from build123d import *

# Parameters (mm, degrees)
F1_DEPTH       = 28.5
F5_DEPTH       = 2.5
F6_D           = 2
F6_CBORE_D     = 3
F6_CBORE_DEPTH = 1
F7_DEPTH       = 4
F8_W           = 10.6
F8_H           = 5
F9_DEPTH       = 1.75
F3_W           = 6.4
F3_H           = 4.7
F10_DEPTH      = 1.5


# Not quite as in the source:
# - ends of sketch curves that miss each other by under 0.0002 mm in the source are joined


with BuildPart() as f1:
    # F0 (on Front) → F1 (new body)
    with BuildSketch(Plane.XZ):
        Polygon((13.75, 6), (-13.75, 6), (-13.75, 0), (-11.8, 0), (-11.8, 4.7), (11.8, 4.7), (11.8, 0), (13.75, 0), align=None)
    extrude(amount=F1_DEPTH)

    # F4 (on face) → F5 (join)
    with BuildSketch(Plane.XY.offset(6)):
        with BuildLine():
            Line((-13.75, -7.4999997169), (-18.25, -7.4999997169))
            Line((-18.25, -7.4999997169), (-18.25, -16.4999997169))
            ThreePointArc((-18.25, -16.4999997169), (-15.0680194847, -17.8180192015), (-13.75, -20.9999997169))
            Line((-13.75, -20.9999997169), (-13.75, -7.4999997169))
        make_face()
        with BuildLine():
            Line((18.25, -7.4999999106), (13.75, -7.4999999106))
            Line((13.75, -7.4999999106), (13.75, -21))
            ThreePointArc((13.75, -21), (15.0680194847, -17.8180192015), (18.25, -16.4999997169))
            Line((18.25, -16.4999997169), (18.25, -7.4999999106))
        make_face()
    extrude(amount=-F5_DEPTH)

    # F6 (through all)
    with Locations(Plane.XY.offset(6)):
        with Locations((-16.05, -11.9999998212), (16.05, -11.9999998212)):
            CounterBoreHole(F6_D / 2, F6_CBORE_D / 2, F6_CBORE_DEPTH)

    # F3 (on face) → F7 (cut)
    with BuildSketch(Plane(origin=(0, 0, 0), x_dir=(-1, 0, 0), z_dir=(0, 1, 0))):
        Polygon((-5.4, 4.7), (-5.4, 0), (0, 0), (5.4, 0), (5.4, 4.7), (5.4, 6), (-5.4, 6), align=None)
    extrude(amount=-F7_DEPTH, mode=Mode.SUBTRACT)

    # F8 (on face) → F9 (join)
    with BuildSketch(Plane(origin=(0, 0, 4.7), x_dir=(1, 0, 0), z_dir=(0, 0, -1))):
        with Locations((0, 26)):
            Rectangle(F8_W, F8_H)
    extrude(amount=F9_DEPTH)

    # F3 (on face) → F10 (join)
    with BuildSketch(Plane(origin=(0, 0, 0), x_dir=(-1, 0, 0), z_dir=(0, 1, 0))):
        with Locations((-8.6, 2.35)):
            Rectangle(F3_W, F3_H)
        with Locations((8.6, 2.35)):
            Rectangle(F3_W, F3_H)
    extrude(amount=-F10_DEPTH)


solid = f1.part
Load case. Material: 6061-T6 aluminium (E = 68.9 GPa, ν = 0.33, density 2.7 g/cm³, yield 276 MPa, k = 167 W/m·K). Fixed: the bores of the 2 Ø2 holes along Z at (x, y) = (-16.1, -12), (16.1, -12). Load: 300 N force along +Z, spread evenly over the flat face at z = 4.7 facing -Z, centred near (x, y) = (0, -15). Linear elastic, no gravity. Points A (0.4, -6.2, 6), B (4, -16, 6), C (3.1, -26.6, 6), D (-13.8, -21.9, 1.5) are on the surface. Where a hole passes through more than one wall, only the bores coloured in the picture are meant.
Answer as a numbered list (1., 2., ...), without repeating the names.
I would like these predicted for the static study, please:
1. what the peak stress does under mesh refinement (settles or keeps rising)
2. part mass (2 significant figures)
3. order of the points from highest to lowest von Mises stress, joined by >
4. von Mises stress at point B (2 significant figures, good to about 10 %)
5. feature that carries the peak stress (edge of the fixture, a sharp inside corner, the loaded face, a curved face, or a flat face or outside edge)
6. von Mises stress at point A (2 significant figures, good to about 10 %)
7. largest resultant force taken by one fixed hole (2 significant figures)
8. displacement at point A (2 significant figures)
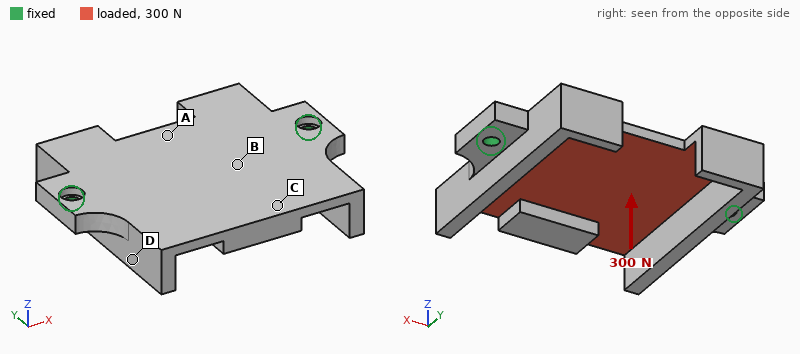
1. keeps rising
2. 5.0 g
3. A > B > C > D
4. 49 MPa
5. edge of the fixture
6. 70 MPa
7. 310 N
8. 61 µm
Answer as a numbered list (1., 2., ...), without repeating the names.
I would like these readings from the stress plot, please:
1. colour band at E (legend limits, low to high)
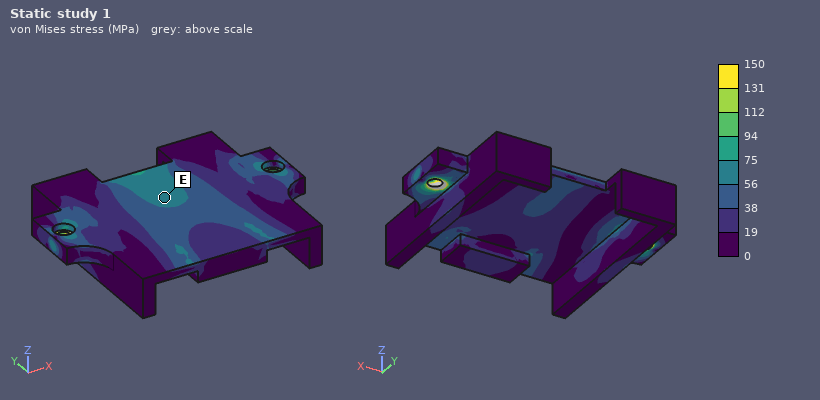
1. 56 to 75 MPa
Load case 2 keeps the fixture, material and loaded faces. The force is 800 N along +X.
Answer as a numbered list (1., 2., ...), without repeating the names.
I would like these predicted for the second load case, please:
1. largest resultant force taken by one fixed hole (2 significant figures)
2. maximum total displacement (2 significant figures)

1. 400 N
2. 13 µm
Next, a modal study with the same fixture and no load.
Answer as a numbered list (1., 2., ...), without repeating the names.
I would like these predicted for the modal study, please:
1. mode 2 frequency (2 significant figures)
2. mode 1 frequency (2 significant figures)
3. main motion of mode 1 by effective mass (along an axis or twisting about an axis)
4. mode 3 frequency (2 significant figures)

1. 7300 Hz
2. 4400 Hz
3. along Z
4. 7500 Hz
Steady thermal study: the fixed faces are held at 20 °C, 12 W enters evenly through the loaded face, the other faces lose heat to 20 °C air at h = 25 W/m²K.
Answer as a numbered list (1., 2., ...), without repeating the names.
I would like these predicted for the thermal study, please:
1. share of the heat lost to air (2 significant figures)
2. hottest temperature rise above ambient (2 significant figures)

1. 4.2 %
2. 15 K
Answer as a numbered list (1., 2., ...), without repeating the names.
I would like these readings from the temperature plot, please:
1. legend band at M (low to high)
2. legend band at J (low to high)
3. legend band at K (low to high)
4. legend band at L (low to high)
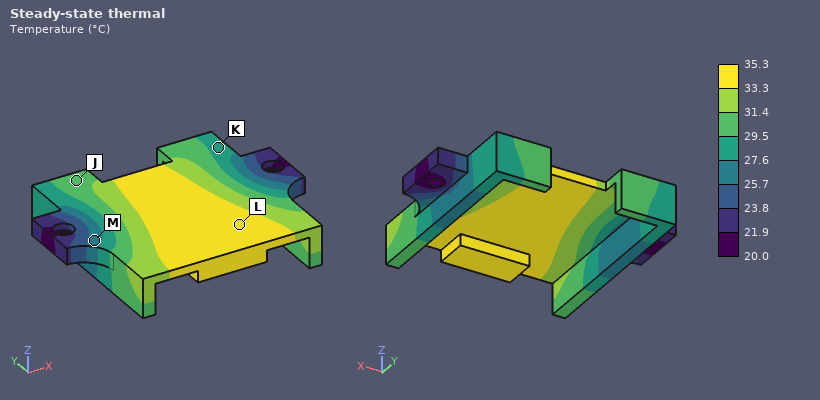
1. 25.7 to 27.6 °C
2. 29.5 to 31.4 °C
3. 27.6 to 29.5 °C
4. 33.3 to 35.3 °C
